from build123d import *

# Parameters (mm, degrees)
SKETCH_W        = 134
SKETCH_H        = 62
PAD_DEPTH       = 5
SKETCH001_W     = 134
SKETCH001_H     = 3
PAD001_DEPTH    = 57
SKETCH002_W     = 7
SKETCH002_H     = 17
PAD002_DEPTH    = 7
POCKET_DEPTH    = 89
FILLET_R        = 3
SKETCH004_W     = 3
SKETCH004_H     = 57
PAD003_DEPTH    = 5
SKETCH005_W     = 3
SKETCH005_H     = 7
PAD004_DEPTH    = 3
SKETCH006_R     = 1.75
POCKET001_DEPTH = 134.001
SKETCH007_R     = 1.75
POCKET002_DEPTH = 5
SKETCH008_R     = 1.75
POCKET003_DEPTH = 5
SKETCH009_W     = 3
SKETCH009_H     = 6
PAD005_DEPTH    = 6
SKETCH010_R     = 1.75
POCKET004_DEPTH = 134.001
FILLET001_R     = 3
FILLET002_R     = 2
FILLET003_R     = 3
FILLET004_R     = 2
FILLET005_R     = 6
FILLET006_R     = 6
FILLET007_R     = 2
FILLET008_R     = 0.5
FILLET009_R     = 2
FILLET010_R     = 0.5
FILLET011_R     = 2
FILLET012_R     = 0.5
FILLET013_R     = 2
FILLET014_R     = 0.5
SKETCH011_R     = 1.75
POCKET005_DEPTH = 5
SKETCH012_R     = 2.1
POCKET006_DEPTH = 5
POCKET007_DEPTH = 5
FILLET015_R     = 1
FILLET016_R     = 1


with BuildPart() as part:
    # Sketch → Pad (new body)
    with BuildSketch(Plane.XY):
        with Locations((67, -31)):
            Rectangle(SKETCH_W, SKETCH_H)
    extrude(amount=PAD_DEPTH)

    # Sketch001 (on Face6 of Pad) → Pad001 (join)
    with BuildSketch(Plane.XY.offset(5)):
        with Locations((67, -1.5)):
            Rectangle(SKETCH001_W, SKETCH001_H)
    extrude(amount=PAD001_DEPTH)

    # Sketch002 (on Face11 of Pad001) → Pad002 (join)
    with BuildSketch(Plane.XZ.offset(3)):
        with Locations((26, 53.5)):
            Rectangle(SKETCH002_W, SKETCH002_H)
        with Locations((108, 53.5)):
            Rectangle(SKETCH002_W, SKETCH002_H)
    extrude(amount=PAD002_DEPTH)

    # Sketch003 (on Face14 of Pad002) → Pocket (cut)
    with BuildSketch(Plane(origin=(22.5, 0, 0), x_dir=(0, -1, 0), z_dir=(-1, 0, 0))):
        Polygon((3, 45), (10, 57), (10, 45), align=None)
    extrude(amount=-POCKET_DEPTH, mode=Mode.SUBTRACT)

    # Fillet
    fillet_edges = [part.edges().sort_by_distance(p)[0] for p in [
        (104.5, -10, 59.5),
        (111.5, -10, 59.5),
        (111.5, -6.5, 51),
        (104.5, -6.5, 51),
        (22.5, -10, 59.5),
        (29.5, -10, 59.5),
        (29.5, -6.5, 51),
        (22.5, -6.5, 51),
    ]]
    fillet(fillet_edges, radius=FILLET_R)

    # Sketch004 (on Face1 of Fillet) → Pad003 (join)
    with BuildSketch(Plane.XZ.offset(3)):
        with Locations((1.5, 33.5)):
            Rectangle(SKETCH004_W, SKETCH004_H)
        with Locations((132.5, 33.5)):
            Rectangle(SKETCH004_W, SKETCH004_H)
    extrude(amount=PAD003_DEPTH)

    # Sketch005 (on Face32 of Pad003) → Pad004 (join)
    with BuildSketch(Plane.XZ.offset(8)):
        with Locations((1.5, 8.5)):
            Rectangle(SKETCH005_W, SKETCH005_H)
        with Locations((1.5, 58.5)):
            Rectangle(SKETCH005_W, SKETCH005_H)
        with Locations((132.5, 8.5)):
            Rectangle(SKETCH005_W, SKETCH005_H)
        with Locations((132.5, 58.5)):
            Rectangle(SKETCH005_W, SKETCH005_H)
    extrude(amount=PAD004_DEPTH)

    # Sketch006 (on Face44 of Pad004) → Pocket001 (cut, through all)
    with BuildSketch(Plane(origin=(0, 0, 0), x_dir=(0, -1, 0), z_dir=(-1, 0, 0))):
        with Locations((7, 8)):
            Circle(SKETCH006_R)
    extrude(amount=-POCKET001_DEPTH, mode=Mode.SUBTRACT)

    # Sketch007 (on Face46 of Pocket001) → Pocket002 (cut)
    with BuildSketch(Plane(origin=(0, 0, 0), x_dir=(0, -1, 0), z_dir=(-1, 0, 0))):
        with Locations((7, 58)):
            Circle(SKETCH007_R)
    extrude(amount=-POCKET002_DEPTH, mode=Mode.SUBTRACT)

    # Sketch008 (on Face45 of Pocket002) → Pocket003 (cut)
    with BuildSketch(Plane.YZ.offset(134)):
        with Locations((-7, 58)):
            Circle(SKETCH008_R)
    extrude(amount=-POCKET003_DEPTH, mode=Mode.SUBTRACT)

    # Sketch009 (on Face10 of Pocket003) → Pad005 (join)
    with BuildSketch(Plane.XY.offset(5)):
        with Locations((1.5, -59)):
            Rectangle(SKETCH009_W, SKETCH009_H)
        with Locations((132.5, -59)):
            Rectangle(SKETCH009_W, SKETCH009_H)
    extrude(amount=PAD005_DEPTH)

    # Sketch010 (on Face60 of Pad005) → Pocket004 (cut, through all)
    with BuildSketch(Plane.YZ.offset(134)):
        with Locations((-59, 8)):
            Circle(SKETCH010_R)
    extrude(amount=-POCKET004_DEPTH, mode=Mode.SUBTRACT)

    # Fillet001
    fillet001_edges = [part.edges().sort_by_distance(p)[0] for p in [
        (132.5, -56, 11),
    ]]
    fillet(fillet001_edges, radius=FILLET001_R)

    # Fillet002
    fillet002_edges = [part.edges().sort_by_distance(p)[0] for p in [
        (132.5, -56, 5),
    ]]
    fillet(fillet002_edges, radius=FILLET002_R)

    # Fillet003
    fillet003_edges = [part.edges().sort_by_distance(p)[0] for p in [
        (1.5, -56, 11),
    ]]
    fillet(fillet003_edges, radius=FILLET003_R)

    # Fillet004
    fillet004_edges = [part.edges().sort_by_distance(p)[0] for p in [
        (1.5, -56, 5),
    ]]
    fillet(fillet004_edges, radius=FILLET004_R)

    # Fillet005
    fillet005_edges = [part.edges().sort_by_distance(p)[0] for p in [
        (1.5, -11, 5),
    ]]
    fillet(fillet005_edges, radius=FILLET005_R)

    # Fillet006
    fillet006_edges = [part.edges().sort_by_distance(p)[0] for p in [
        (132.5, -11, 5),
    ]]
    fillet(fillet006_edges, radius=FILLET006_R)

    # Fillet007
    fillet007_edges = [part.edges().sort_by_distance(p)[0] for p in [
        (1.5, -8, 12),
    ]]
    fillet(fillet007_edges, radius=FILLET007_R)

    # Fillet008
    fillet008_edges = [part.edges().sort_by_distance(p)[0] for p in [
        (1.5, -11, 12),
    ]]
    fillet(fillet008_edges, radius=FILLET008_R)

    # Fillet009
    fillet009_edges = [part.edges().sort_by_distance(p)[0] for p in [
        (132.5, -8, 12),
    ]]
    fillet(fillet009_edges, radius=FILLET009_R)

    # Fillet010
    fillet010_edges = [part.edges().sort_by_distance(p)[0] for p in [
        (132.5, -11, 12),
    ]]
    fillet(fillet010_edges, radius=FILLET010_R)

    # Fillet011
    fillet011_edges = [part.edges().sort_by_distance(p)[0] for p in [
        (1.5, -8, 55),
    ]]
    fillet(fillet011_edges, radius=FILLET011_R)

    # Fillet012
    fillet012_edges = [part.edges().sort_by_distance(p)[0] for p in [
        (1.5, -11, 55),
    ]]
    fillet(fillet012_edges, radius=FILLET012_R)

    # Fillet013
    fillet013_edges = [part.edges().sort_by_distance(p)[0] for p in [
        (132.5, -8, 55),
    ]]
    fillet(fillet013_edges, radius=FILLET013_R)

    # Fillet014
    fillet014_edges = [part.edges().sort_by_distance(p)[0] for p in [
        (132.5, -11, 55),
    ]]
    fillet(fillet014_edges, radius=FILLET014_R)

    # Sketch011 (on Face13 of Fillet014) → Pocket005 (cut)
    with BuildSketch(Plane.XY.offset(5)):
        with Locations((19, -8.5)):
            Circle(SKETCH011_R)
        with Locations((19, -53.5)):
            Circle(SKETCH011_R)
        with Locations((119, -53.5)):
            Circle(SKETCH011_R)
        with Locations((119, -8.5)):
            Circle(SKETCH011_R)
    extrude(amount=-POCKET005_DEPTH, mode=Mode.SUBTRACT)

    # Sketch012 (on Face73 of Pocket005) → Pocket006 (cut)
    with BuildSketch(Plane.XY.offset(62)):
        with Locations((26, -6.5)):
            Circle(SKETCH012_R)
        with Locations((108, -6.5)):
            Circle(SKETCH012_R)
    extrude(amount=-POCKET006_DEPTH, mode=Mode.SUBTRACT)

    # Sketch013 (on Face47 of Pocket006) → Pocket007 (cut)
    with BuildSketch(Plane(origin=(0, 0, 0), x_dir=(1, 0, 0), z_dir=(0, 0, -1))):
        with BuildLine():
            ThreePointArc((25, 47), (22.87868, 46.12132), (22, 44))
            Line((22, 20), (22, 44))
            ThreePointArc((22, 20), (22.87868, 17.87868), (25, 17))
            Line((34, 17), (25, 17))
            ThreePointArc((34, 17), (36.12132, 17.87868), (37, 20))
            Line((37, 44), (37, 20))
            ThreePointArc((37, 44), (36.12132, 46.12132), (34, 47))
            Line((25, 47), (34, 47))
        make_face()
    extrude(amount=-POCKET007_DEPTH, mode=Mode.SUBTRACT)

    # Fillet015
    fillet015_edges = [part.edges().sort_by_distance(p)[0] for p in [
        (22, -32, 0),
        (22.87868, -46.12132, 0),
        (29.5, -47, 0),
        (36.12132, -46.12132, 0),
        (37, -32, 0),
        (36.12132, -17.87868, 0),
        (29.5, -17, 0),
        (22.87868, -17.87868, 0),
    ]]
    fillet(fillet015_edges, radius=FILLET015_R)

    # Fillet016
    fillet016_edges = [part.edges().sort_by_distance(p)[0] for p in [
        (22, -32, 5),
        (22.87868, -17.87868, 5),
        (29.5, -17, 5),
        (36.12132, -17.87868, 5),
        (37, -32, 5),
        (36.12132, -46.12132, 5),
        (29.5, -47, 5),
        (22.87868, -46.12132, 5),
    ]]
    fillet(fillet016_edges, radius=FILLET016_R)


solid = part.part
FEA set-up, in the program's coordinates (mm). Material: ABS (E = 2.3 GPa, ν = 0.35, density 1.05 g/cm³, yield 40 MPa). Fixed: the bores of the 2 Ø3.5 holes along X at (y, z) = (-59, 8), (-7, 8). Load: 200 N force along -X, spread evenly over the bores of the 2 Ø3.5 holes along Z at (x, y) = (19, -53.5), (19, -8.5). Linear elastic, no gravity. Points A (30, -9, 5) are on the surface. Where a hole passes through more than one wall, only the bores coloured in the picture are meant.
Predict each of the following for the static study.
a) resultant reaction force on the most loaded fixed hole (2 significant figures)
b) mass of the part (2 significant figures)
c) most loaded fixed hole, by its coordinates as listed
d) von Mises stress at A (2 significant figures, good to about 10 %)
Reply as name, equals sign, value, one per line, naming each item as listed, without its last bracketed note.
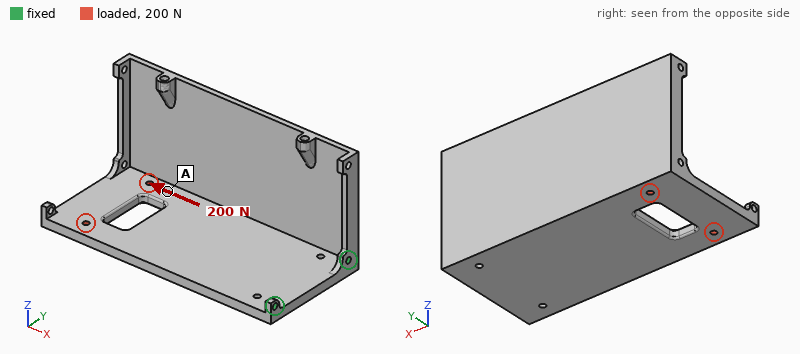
resultant reaction force on the most loaded fixed hole = 110 N
mass of the part = 68 g
most loaded fixed hole, by its coordinates as listed = (-7, 8)
von Mises stress at A = 1.0 MPa
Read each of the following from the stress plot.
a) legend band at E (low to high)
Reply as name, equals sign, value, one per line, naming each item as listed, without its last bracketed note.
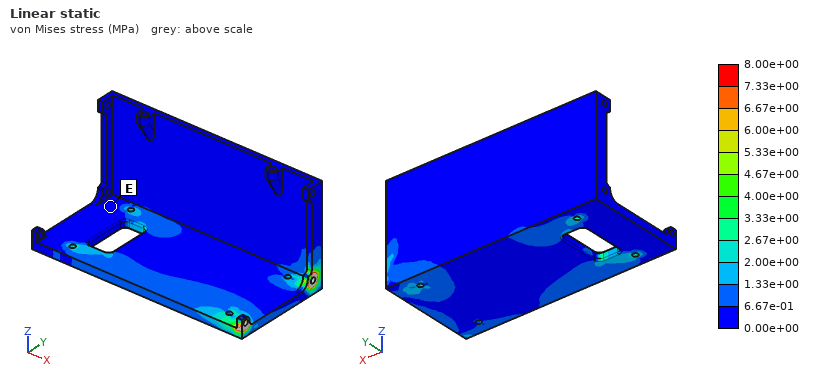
legend band at E = 0.00e+00 to 6.67e-01 MPa
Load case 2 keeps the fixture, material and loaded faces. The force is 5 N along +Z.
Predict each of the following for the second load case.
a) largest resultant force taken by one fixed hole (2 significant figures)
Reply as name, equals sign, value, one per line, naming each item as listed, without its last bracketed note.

largest resultant force taken by one fixed hole = 3.7 N
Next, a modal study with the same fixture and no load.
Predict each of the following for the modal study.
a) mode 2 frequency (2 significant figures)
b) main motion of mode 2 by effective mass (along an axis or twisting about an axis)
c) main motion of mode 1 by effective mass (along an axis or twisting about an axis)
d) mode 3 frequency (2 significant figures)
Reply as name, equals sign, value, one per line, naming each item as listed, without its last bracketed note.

mode 2 frequency = 130 Hz
main motion of mode 2 by effective mass = along Y
main motion of mode 1 by effective mass = along Z
mode 3 frequency = 320 Hz
